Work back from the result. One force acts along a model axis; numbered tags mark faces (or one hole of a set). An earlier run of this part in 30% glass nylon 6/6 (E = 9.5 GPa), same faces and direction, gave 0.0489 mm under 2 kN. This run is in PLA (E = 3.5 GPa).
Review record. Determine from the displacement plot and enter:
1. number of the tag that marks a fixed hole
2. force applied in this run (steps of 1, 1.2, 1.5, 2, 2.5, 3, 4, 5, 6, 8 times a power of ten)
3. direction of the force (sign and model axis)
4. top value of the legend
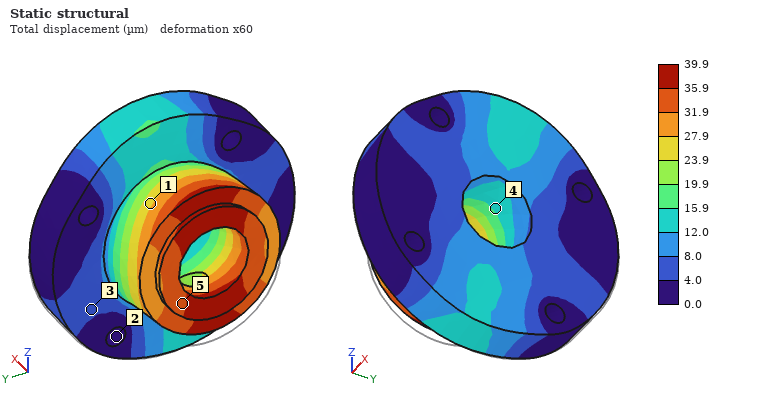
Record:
2
600 N
+Z
39.9 µm
